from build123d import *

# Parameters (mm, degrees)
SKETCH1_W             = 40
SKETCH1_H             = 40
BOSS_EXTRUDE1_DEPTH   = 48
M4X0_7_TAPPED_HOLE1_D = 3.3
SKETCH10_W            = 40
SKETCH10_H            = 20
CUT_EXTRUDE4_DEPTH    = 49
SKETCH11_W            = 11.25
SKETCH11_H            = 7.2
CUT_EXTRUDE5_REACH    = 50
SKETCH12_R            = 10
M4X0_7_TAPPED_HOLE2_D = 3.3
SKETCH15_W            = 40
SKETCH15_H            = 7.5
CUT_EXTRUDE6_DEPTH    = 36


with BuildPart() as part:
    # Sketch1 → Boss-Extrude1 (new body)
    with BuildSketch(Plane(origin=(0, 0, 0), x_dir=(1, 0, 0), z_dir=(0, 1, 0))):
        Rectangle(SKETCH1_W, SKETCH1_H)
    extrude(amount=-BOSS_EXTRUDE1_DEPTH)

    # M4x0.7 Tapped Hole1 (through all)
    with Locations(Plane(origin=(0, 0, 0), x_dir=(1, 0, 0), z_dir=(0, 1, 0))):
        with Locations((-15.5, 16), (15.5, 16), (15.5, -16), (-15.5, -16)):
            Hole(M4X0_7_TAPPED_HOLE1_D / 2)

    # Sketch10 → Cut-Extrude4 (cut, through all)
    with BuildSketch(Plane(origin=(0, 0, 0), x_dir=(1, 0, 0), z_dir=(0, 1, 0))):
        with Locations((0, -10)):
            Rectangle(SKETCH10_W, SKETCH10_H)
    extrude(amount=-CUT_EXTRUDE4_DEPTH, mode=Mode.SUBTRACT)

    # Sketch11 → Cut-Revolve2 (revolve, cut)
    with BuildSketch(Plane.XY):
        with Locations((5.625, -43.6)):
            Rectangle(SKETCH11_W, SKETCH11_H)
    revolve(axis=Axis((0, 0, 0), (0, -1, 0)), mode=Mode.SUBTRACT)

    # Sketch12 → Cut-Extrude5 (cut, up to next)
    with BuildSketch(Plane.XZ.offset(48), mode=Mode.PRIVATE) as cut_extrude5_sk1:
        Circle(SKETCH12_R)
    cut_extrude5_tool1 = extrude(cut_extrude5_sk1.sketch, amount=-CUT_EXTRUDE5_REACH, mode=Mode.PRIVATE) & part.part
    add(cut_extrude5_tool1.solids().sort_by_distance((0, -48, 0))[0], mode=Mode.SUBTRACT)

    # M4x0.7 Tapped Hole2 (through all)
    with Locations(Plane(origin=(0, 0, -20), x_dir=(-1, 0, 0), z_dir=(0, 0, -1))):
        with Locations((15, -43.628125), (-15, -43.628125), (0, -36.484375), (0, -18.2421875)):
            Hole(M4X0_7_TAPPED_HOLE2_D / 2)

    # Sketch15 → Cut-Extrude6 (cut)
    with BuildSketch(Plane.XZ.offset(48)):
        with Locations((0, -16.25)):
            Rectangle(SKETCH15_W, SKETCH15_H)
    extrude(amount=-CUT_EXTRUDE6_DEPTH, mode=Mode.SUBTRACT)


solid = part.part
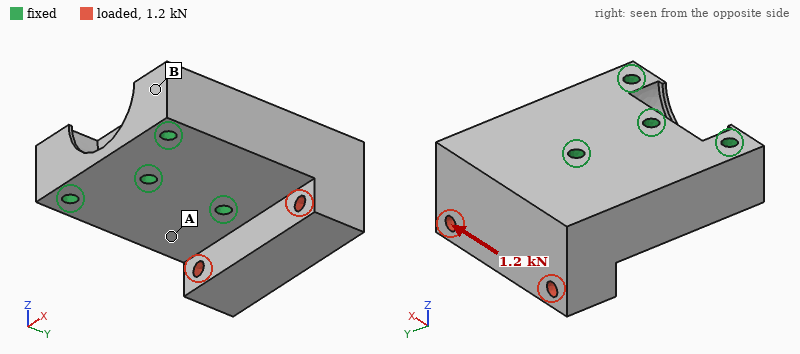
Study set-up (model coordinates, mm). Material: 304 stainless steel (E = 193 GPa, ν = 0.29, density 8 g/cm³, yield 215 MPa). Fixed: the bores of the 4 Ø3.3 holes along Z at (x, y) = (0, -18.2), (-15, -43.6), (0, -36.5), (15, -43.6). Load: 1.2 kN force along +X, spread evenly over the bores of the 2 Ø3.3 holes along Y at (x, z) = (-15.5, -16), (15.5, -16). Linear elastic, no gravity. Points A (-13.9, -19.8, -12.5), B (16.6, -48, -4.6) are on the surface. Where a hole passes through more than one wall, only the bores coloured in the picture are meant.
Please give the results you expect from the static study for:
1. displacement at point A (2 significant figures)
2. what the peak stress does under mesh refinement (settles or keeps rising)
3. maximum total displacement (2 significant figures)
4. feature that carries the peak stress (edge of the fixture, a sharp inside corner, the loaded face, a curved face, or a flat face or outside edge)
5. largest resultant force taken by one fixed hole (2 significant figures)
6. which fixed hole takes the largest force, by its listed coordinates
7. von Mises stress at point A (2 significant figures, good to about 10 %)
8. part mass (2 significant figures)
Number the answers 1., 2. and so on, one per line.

1. 1.0 µm
2. keeps rising
3. 3.7 µm
4. edge of the fixture
5. 1.4 kN
6. (0, -18.2)
7. 6.9 MPa
8. 200 g
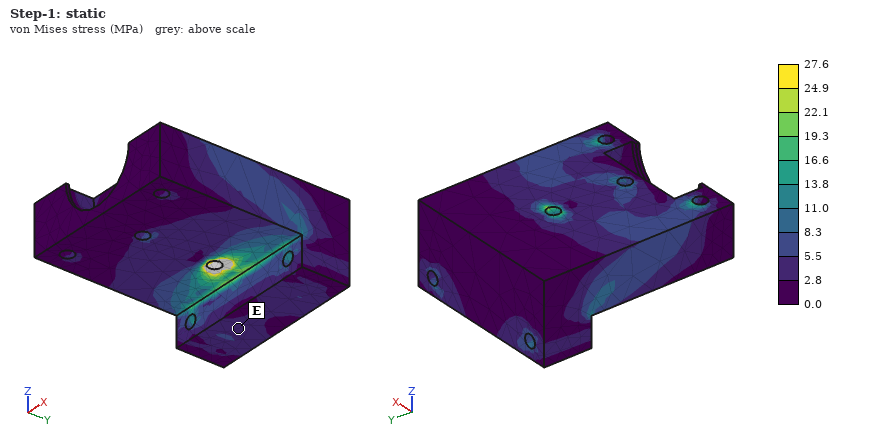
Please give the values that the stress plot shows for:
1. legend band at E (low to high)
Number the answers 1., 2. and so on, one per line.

1. 2.8 to 5.5 MPa
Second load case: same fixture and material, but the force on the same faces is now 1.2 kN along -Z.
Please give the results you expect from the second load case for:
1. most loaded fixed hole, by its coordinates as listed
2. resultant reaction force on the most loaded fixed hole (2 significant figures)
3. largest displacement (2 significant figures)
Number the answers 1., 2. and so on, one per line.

1. (0, -18.2)
2. 1.4 kN
3. 4.1 µm
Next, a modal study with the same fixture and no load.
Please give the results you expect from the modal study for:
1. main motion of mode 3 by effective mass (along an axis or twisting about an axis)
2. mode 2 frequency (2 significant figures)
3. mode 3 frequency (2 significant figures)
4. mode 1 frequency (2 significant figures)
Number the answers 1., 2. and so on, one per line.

1. along X
2. 12 kHz
3. 18 kHz
4. 12 kHz
